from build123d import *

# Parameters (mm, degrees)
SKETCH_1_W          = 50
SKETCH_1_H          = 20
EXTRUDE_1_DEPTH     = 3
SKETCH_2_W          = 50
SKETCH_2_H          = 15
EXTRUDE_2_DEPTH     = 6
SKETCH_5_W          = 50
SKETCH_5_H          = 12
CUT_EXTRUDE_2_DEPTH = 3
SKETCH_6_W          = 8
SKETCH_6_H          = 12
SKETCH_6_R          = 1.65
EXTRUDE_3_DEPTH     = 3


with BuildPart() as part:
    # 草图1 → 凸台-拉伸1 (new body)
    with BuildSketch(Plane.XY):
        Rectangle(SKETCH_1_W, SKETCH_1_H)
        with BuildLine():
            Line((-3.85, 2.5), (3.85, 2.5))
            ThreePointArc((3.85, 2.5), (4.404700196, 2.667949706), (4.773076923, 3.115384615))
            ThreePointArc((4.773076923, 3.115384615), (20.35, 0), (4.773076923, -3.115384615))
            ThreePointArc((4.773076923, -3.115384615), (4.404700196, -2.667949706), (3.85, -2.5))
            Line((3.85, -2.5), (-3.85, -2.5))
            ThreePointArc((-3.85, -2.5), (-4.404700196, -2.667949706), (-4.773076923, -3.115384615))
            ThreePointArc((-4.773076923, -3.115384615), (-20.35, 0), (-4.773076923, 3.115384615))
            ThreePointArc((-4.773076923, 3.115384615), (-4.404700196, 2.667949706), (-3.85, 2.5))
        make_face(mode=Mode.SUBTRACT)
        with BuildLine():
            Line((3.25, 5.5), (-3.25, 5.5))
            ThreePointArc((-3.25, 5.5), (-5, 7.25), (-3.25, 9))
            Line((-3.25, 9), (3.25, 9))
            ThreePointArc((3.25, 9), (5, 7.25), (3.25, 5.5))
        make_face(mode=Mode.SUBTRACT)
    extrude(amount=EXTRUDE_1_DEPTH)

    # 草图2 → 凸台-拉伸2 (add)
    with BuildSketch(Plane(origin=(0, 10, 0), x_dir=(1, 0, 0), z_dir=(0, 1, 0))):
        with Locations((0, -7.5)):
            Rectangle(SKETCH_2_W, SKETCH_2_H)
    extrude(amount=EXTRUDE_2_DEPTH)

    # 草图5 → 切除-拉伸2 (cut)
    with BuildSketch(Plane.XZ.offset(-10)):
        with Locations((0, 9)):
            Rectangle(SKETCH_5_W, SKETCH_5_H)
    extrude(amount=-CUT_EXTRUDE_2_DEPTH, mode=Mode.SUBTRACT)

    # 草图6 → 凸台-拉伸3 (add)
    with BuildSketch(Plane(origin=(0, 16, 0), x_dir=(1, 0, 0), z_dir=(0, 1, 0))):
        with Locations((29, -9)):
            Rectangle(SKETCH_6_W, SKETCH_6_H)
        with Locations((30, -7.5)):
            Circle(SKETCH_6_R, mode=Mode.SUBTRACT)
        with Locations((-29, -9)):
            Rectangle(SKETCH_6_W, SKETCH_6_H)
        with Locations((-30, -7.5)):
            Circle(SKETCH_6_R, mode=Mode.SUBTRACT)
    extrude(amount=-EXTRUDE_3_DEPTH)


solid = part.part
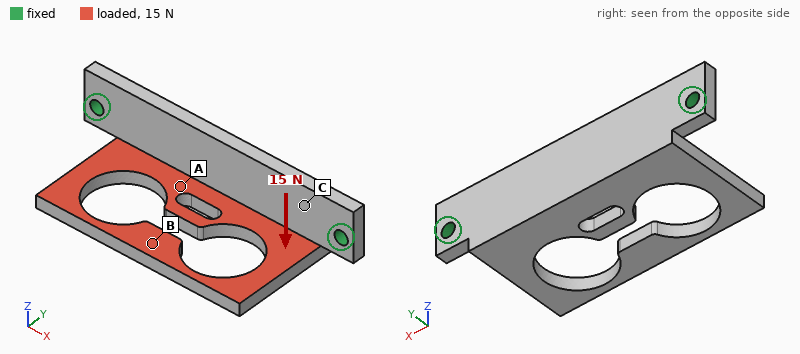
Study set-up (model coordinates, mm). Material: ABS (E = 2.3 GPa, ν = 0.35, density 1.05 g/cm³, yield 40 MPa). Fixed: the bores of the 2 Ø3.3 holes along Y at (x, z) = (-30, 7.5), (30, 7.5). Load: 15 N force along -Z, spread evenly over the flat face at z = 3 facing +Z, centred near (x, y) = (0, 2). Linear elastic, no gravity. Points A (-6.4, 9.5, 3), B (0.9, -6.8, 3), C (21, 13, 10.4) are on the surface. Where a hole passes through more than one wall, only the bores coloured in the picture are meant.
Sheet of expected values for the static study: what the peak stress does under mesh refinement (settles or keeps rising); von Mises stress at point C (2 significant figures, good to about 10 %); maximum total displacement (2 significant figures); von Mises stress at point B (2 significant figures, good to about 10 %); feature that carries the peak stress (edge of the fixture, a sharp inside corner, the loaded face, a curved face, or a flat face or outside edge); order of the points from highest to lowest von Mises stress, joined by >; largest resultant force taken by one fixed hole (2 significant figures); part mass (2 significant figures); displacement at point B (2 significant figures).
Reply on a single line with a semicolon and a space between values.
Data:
keeps rising; 2.8 MPa; 0.73 mm; 1.5 MPa; edge of the fixture; C > B > A; 7.5 N; 5.0 g; 0.64 mm
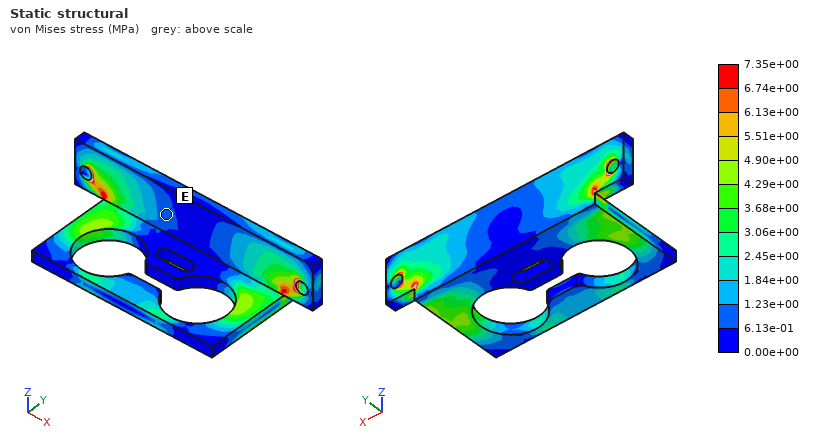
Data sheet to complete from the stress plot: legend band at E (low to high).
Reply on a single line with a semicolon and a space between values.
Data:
6.13e-01 to 1.23e+00 MPa
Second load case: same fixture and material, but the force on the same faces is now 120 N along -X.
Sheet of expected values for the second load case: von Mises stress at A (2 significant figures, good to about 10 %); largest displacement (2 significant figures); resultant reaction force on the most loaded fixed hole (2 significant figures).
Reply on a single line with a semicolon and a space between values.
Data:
3.9 MPa; 0.72 mm; 67 N
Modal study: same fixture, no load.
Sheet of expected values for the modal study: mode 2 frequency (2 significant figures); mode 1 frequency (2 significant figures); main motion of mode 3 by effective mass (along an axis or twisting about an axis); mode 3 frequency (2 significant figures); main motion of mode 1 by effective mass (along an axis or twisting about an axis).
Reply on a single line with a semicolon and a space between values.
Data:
1200 Hz; 590 Hz; along Y; 1700 Hz; along Z
